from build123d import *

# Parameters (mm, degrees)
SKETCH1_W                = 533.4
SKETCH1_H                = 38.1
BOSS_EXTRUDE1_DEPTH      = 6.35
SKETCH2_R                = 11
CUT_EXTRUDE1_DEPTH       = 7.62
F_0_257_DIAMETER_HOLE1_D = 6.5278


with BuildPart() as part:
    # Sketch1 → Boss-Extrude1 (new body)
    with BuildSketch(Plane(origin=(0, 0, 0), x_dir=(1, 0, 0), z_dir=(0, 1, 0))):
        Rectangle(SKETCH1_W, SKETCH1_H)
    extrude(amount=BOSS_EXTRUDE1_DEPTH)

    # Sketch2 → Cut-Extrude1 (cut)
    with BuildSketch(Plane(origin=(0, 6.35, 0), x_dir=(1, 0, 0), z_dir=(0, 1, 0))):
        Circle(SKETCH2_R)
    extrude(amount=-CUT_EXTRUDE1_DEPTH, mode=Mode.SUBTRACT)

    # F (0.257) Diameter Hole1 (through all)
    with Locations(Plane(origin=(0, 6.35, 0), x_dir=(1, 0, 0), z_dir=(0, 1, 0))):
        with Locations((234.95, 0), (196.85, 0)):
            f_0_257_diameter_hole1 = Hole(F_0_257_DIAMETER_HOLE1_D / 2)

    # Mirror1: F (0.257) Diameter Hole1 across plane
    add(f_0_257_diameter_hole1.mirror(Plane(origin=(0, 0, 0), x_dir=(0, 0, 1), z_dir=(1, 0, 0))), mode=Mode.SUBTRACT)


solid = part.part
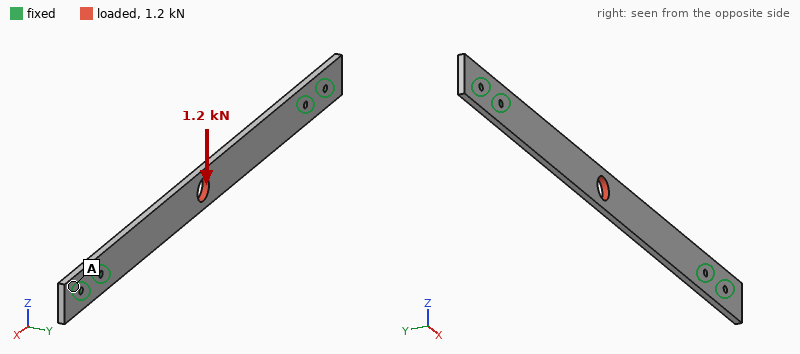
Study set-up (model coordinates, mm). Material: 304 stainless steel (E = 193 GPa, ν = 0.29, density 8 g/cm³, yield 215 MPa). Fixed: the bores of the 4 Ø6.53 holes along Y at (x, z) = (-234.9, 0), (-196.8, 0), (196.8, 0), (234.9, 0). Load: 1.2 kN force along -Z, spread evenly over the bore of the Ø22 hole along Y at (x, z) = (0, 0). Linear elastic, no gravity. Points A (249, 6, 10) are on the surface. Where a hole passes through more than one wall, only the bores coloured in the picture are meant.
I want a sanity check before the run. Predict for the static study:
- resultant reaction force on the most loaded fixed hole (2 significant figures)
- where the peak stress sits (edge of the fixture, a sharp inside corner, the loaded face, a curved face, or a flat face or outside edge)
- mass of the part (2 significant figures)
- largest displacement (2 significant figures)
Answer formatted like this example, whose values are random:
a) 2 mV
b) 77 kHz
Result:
a) 1.7 kN
b) edge of the fixture
c) 1.0 kg
d) 94 µm
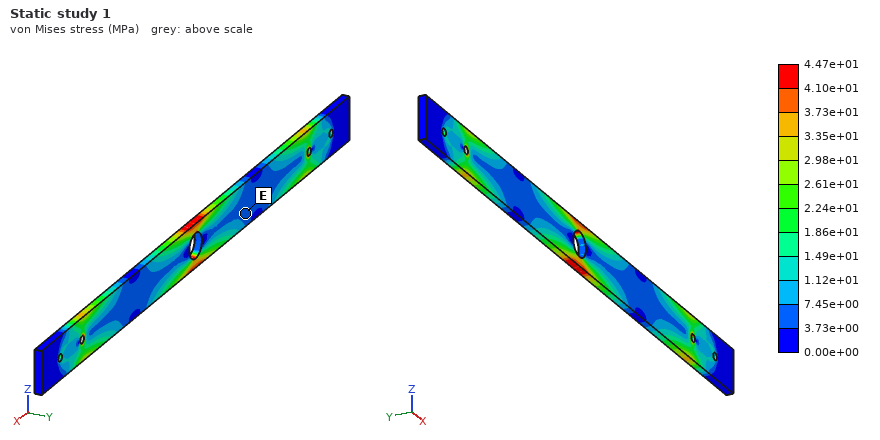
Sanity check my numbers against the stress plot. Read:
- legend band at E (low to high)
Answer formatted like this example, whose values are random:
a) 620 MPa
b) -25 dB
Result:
a) 3.73e+00 to 7.45e+00 MPa
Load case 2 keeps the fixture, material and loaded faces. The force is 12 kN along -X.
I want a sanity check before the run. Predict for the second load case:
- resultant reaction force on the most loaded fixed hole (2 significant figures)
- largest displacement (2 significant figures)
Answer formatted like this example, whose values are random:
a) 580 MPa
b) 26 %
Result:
a) 4.9 kN
b) 26 µm
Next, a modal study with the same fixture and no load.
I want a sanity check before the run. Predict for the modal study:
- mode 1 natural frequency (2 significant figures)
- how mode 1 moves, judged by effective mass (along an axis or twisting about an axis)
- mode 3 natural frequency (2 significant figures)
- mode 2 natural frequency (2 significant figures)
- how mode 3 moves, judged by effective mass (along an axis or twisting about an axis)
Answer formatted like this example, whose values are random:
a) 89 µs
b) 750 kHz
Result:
a) 200 Hz
b) along Y
c) 1000 Hz
d) 570 Hz
e) along Z
